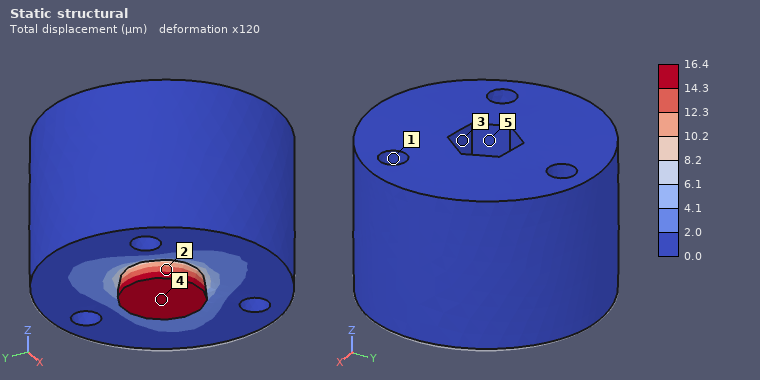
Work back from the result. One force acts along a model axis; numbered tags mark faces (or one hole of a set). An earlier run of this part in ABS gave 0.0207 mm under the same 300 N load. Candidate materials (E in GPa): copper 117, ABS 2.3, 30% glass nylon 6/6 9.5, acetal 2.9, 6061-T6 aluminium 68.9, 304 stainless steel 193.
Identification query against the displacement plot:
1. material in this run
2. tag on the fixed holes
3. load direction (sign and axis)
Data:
acetal
1
+Z
